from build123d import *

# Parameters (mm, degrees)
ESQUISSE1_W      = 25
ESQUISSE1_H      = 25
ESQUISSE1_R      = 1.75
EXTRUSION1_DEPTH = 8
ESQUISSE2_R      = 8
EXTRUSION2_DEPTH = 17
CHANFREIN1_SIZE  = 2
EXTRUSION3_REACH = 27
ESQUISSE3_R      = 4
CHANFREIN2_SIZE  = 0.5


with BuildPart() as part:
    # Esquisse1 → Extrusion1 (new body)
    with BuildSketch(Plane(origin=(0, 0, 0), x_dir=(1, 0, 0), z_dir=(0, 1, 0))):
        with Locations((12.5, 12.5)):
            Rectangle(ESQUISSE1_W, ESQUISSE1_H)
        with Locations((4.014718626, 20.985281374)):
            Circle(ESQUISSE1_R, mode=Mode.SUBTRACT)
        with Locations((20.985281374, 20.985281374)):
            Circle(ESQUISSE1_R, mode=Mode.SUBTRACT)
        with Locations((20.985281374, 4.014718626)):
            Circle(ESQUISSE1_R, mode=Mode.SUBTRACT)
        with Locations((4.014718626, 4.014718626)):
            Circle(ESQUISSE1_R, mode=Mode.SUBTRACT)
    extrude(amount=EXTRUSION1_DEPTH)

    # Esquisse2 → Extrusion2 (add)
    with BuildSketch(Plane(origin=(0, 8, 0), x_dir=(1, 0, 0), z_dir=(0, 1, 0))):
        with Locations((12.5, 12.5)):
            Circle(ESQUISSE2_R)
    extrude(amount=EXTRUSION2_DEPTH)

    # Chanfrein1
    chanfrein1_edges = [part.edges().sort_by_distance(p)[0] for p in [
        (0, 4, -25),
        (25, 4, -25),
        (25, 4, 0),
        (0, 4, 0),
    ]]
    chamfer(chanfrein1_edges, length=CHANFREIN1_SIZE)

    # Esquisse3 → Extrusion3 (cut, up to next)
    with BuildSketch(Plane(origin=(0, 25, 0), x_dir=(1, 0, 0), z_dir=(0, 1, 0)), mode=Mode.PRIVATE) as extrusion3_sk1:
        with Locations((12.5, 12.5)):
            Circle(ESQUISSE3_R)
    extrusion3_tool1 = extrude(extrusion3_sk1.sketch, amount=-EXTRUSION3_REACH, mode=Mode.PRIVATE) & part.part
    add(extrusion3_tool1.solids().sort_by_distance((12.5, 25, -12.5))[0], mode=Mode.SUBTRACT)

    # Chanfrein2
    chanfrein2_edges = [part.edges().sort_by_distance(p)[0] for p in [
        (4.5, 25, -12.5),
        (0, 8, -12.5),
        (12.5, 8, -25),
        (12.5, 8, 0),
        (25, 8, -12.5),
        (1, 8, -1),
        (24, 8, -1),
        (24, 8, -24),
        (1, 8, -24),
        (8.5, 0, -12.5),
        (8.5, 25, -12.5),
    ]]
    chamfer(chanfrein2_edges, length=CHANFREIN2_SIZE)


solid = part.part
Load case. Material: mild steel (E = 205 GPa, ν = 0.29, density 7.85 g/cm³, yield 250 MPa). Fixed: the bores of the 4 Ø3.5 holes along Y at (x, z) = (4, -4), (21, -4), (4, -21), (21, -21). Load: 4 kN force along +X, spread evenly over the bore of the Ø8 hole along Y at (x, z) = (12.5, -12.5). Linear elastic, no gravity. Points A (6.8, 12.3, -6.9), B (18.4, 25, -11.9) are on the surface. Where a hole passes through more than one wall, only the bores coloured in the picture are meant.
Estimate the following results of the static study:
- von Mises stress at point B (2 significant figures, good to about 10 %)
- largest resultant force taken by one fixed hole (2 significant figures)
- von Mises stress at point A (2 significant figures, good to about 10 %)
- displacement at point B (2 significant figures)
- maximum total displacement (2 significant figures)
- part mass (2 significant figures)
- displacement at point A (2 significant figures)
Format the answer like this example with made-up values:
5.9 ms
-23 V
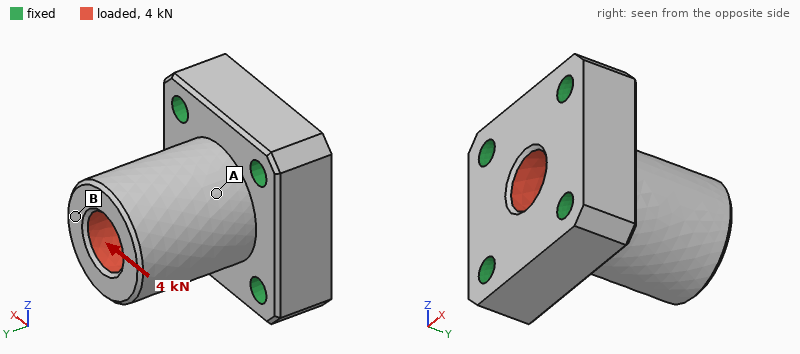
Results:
11 MPa
1.5 kN
29 MPa
10.0 µm
10 µm
53 g
3.8 µm
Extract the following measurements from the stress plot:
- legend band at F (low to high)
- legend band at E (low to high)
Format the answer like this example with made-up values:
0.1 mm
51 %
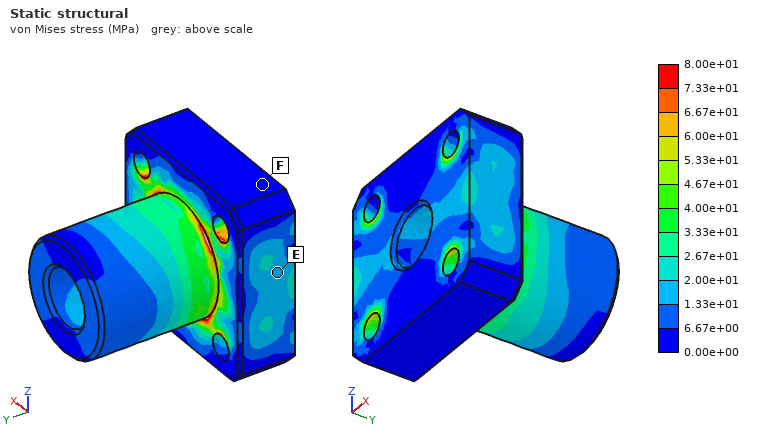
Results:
0.00e+00 to 6.67e+00 MPa
1.33e+01 to 2.00e+01 MPa
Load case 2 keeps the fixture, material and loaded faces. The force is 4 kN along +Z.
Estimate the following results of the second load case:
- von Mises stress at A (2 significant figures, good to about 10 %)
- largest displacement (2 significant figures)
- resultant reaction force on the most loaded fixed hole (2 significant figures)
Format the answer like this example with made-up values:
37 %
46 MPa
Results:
30 MPa
10 µm
1.5 kN
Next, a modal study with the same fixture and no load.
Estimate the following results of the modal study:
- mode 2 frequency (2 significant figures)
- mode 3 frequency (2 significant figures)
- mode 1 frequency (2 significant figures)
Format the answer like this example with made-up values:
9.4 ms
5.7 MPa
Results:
22 kHz
42 kHz
22 kHz
